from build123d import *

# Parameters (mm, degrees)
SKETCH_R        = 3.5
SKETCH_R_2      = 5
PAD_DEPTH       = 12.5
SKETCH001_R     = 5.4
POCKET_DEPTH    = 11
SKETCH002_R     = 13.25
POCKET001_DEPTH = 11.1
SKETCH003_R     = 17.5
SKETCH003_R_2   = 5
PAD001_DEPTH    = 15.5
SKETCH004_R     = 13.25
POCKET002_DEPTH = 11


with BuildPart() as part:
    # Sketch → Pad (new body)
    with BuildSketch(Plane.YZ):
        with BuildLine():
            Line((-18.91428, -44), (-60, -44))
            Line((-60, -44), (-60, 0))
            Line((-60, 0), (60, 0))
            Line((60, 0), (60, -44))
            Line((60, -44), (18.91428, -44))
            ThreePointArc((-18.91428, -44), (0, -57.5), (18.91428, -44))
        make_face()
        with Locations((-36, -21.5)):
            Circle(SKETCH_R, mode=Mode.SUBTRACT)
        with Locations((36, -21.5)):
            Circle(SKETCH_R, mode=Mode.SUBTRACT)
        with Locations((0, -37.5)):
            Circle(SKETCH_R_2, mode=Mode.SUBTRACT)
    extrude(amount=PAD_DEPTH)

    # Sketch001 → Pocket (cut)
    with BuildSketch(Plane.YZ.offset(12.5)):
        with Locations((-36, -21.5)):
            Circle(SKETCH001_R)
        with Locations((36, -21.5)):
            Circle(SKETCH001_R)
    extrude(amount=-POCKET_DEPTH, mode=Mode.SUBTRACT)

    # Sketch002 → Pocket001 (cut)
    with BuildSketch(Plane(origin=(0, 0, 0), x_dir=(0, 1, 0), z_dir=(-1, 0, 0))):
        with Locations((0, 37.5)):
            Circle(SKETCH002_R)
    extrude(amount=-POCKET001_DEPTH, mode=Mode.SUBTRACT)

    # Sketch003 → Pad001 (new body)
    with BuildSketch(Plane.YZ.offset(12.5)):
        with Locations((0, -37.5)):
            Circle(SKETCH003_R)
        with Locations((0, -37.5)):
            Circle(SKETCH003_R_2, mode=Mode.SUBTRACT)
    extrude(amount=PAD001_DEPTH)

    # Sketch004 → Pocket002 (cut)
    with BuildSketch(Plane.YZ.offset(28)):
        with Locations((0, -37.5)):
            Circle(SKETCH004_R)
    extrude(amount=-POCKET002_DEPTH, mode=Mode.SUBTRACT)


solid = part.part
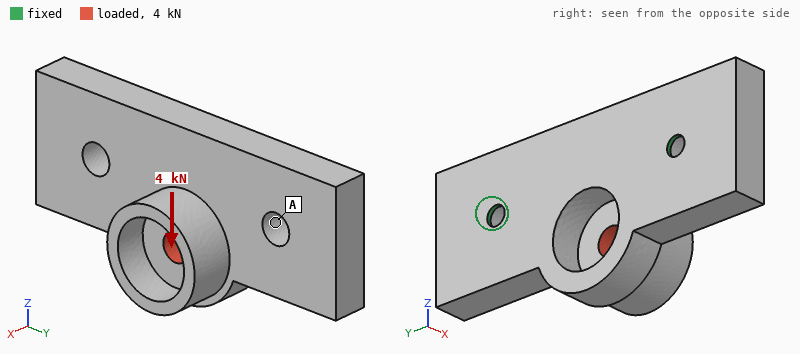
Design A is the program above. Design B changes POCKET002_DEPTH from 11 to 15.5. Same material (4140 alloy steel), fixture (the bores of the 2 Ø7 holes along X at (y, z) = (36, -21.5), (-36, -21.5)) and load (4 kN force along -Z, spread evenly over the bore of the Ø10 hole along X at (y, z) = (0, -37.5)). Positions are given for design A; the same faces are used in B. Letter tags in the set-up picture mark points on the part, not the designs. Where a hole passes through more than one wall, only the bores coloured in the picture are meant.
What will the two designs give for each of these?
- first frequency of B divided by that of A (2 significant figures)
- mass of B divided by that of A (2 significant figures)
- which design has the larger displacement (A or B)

1.0
0.97
A
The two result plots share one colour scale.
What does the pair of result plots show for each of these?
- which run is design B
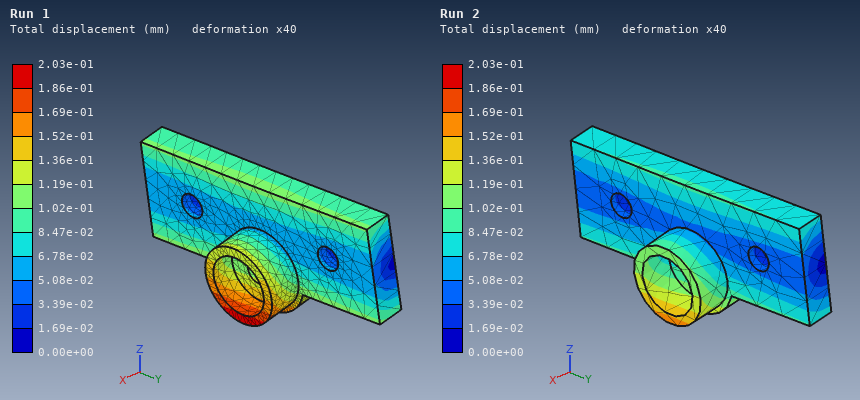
Run 2
